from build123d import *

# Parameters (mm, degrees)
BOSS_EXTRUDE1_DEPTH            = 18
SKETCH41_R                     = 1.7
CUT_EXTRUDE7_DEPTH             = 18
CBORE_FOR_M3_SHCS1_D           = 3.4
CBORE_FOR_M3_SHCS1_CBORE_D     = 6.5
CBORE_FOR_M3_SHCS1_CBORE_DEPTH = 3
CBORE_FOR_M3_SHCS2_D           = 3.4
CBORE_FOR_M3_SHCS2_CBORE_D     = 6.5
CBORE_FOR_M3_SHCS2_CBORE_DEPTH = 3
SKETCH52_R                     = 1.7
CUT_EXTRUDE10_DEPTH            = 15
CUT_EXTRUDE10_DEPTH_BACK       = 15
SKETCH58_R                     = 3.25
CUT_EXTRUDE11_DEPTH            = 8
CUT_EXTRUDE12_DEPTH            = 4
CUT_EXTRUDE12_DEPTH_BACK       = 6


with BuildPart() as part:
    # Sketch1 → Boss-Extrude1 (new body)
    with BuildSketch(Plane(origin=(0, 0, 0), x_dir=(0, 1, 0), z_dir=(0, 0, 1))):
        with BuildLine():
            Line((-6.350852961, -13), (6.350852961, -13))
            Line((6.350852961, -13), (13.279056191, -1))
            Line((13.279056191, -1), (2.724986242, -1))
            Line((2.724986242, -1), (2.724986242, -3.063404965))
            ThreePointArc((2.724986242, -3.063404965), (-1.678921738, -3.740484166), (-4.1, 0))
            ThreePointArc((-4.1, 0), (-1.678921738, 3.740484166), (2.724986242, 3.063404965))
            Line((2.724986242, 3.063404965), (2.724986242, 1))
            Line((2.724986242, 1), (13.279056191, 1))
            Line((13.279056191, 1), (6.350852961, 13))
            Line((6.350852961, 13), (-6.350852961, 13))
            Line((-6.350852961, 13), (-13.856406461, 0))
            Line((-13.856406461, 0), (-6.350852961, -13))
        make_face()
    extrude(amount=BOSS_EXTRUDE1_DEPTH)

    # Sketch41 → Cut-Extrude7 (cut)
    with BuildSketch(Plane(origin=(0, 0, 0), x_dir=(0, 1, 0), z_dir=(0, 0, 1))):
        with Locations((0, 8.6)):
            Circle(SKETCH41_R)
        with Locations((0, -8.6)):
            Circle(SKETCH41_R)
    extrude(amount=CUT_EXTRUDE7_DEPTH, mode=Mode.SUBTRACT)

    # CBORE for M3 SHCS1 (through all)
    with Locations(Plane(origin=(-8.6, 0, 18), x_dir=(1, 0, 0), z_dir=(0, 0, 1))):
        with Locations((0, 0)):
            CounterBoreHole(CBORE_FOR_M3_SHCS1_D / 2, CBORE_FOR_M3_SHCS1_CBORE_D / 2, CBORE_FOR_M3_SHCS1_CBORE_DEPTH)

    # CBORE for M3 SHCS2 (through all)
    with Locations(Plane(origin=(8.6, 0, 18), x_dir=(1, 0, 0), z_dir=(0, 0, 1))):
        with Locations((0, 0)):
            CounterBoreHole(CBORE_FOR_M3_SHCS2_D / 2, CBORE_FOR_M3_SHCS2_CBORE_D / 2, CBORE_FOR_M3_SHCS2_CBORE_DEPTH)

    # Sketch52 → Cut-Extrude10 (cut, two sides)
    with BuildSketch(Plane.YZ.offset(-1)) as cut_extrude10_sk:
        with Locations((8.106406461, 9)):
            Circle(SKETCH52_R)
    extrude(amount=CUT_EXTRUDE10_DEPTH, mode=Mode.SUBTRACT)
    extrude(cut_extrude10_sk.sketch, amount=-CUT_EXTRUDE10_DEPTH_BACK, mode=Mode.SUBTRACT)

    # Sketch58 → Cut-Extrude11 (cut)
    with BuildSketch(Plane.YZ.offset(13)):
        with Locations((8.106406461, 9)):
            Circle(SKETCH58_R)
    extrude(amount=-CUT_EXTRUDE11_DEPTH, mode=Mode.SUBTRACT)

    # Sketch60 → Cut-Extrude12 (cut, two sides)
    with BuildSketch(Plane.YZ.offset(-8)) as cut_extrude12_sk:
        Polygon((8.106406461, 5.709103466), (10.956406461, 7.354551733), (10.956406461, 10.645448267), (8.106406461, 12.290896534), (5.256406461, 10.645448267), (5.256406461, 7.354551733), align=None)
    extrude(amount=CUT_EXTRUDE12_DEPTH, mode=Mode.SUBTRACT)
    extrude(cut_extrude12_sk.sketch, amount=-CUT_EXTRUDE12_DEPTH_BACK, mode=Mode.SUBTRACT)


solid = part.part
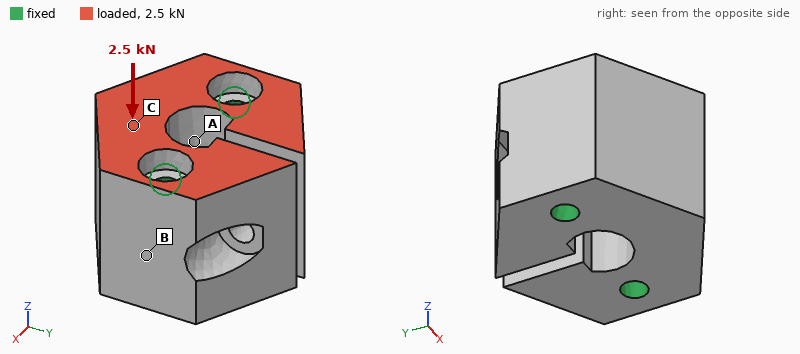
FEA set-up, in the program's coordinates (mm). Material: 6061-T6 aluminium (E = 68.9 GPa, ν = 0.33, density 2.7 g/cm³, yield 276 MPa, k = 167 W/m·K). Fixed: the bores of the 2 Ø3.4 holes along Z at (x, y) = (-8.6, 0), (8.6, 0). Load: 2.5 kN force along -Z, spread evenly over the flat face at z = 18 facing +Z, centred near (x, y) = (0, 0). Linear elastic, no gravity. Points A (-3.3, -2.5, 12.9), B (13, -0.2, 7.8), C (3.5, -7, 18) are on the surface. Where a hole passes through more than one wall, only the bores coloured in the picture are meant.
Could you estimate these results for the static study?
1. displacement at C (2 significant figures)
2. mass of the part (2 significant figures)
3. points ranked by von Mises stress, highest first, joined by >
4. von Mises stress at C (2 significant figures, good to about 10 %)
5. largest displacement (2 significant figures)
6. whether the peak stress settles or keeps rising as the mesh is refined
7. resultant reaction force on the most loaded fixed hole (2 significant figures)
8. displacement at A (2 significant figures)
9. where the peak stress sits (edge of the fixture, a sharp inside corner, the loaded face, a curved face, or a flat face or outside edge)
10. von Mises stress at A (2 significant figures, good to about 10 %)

2.4 µm
20 g
A > C > B
6.7 MPa
4.3 µm
keeps rising
1.3 kN
1.1 µm
edge of the fixture
8.9 MPa
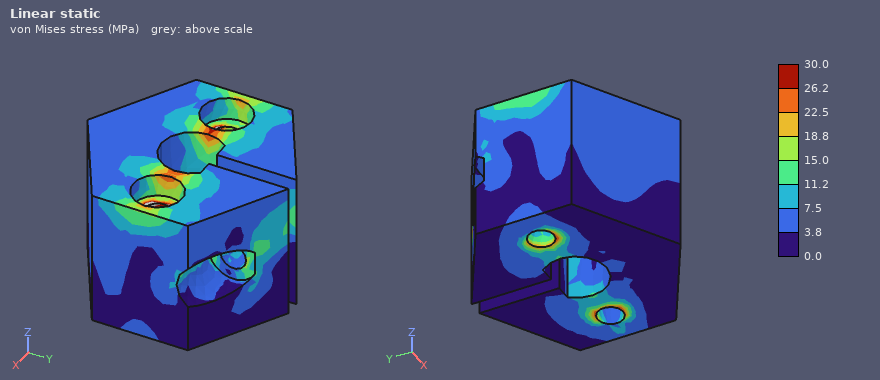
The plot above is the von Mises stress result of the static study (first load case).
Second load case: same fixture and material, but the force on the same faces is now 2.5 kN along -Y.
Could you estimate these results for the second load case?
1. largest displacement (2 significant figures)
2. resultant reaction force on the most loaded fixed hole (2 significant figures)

12 µm
1.3 kN
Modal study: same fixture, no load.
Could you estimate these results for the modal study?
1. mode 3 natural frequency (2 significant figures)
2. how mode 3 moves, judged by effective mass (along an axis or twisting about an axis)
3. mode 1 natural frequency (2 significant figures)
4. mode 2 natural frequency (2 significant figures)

39 kHz
twisting about X
32 kHz
33 kHz
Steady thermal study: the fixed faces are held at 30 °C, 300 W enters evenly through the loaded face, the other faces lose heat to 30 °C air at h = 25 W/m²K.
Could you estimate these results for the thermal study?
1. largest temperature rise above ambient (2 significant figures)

55 K
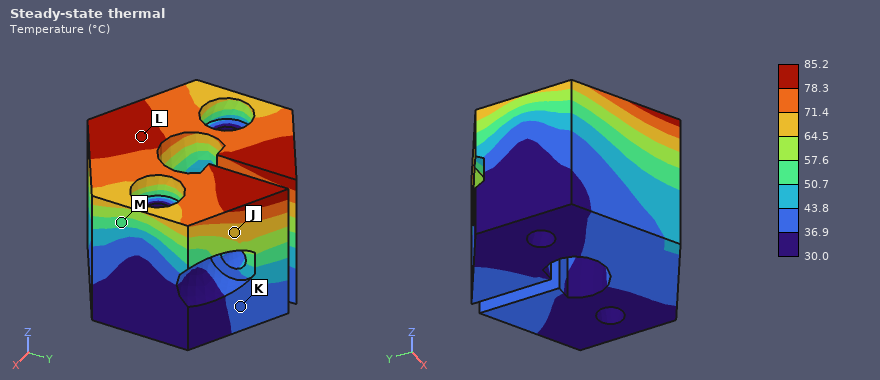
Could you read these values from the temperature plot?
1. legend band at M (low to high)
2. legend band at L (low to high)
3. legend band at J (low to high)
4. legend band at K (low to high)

50.7 to 57.6 °C
78.3 to 85.2 °C
64.5 to 71.4 °C
36.9 to 43.8 °C
